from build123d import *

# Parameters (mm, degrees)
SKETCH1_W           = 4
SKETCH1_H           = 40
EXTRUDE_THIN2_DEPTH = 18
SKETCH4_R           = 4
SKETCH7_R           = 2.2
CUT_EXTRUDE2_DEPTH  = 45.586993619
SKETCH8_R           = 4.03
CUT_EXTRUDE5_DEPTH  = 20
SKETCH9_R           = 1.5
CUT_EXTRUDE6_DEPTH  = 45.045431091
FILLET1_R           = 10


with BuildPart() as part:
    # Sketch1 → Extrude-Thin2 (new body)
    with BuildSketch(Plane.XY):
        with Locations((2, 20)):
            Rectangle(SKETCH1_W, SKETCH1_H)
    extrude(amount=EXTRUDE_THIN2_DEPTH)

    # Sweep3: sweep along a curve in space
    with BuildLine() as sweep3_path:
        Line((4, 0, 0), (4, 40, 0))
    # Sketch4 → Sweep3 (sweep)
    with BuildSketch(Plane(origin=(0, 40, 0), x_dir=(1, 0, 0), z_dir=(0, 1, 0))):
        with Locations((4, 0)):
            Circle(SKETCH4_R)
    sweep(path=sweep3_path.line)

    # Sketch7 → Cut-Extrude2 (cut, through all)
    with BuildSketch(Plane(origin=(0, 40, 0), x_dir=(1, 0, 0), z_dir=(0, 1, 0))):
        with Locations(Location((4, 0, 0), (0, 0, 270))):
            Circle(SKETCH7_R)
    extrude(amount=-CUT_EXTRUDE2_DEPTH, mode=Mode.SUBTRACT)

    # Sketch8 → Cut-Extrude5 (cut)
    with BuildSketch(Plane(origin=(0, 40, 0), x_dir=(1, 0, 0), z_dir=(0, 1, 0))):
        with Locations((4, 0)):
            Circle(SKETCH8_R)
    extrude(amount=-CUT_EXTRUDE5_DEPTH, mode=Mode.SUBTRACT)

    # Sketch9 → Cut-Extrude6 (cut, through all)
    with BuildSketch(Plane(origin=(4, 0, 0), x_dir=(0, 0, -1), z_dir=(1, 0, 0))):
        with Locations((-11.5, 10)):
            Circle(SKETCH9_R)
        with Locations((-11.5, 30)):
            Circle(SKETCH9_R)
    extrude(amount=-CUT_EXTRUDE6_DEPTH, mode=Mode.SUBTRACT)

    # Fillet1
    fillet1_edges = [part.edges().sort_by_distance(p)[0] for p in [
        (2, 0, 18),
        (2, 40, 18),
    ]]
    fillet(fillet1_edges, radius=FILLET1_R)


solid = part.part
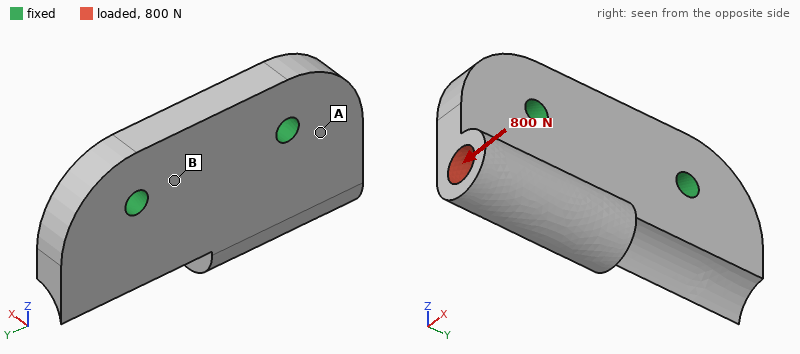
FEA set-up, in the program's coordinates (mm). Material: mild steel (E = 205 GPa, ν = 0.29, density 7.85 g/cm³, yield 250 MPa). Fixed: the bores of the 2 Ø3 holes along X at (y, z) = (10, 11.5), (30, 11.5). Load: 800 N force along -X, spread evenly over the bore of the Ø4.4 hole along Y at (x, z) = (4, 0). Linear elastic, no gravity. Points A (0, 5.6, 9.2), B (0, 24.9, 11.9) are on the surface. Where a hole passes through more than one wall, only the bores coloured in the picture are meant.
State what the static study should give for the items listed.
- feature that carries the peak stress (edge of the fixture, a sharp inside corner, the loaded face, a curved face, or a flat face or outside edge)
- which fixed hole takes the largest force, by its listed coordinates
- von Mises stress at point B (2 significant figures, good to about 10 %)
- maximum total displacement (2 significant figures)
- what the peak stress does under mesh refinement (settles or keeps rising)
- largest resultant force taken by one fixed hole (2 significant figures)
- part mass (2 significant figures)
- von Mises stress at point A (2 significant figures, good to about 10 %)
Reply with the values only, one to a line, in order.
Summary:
edge of the fixture
(10, 11.5)
35 MPa
37 µm
keeps rising
760 N
22 g
93 MPa
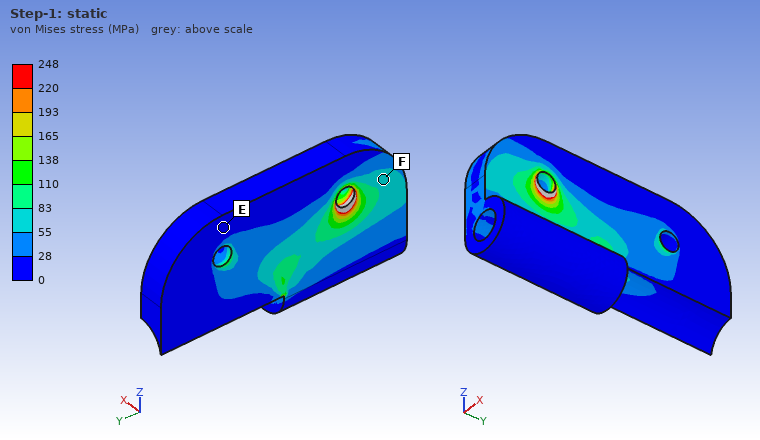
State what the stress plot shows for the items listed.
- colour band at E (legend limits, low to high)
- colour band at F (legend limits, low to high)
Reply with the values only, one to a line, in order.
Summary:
0 to 28 MPa
55 to 83 MPa
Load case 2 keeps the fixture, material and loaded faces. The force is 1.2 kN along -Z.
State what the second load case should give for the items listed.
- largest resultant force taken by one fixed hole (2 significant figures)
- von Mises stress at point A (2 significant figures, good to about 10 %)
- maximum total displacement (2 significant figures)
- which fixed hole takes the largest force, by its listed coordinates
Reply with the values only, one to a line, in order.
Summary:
1.2 kN
18 MPa
14 µm
(10, 11.5)
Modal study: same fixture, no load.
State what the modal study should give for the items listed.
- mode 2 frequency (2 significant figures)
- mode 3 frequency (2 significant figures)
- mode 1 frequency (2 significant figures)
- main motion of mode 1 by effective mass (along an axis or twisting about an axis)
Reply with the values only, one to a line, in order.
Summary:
20 kHz
28 kHz
11 kHz
along X
